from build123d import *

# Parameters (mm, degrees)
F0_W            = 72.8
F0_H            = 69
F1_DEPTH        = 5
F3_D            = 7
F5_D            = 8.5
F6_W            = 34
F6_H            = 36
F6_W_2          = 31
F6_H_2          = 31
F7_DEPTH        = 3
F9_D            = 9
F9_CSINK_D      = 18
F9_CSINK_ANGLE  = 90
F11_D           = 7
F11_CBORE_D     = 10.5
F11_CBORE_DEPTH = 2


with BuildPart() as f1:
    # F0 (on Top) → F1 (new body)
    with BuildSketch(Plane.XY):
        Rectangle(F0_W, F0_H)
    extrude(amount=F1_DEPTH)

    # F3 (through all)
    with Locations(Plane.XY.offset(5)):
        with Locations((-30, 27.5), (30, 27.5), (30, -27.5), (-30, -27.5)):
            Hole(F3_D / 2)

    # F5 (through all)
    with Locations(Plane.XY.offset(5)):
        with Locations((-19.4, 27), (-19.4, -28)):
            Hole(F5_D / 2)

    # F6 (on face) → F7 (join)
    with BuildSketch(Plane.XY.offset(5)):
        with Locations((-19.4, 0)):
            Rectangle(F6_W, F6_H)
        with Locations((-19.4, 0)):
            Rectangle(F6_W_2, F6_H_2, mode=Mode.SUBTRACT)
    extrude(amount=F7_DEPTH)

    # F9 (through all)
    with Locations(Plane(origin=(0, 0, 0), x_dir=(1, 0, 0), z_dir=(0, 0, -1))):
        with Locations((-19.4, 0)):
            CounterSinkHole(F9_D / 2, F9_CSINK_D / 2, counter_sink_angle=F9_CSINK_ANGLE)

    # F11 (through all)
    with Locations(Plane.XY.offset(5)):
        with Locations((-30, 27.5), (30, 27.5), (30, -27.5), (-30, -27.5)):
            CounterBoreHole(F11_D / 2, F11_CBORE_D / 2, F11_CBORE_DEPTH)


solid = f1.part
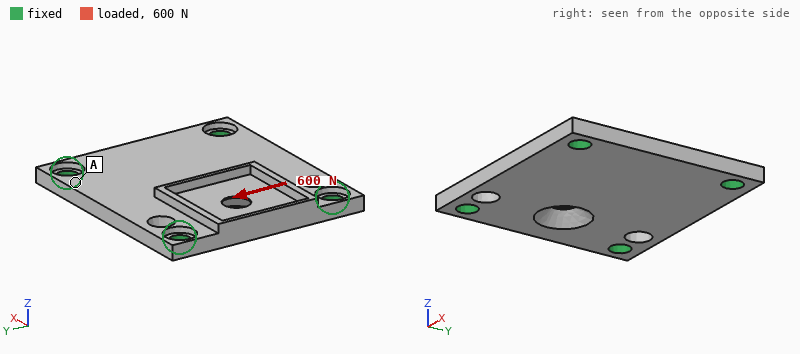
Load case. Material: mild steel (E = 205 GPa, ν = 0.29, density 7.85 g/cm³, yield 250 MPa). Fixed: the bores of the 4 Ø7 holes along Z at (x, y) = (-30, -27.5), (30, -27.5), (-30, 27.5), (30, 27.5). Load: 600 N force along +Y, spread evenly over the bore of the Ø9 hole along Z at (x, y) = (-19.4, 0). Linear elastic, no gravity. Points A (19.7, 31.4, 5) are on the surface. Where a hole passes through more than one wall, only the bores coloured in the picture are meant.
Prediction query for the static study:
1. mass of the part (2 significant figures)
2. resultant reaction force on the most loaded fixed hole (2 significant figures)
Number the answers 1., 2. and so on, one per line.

1. 180 g
2. 240 N
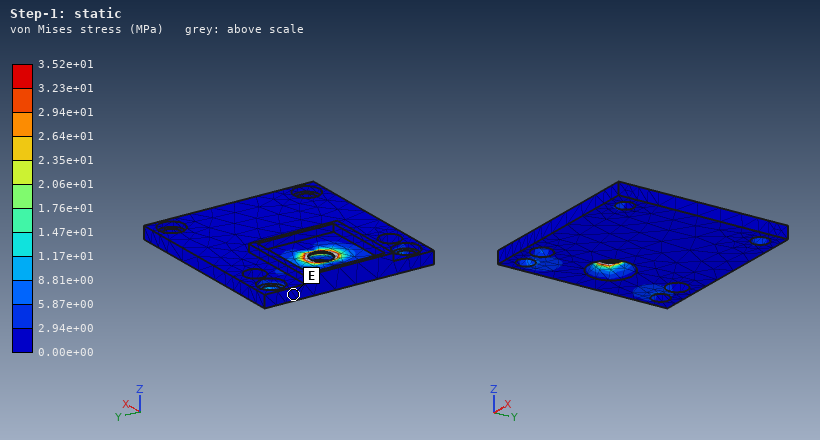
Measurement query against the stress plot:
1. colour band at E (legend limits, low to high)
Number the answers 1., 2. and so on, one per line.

1. 0.00e+00 to 2.94e+00 MPa
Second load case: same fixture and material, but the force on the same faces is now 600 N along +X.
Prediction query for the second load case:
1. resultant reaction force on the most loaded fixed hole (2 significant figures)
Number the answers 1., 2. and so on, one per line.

1. 180 N
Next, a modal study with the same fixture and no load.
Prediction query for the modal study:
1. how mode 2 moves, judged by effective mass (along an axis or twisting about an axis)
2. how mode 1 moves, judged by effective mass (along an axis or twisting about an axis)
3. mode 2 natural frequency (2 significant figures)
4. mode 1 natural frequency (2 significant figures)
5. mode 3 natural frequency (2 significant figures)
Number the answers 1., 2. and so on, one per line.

1. twisting about X
2. along Z
3. 7400 Hz
4. 4900 Hz
5. 8600 Hz
